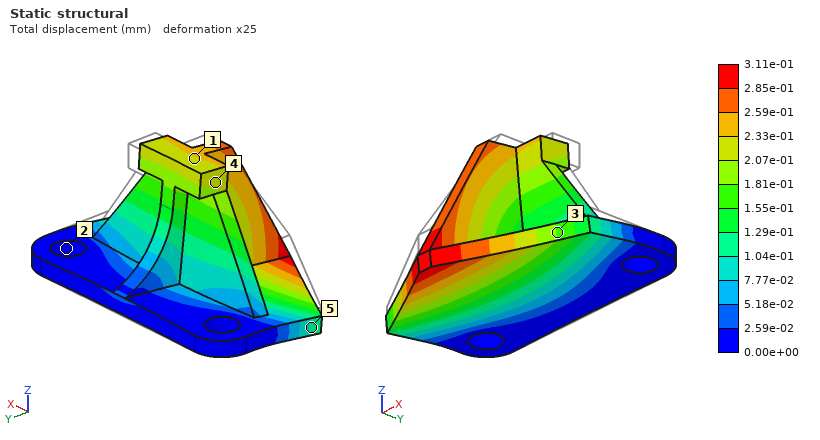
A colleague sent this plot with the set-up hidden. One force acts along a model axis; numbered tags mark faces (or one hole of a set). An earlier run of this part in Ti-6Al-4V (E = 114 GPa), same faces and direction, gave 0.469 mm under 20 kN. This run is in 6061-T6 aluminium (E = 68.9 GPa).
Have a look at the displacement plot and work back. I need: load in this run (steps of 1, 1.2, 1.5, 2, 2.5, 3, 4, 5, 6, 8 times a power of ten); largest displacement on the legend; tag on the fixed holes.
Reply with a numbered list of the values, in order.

1. 8 kN
2. 3.11e-01 mm
3. 2
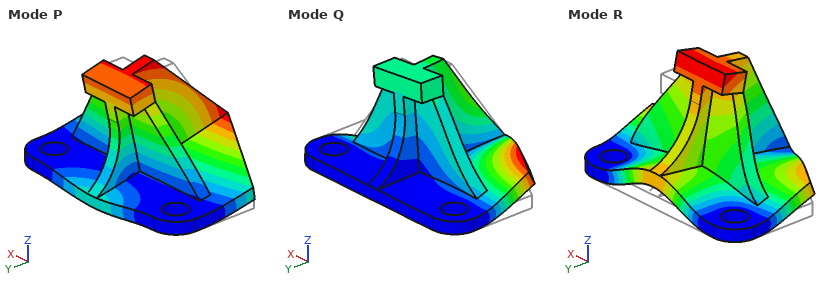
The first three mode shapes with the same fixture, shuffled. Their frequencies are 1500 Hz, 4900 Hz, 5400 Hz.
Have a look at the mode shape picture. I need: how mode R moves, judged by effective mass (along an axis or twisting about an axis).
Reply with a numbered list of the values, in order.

1. along Z
